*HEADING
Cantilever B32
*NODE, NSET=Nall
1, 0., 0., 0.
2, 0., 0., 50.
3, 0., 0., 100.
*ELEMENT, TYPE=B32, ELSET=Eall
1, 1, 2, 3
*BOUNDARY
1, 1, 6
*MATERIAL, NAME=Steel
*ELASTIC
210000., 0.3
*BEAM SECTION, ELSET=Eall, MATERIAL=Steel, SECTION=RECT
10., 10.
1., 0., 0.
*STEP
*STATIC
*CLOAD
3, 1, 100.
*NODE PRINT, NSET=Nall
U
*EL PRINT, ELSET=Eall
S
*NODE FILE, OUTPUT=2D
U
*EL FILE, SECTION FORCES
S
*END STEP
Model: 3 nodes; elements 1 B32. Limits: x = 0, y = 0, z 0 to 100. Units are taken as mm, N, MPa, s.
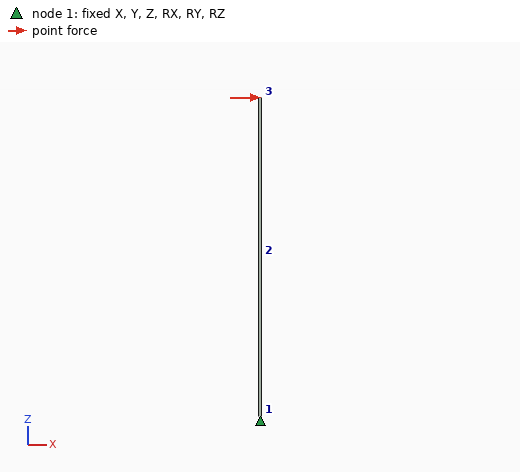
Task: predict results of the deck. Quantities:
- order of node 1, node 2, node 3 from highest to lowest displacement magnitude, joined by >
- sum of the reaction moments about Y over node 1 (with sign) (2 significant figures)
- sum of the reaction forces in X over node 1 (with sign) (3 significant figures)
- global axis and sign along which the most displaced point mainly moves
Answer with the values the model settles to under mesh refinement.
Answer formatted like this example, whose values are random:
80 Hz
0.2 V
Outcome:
node 3 > node 2 > node 1
-10000 N·mm
-100 N
+X
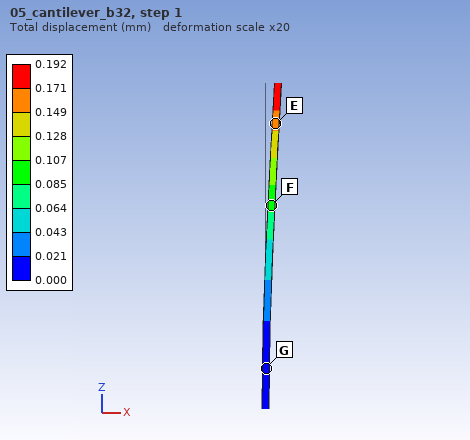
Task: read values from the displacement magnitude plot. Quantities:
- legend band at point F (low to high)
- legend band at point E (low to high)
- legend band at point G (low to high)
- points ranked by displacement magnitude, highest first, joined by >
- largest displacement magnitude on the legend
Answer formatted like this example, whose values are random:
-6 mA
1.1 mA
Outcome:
0.085 to 0.107 mm
0.149 to 0.171 mm
0.000 to 0.021 mm
E > F > G
0.192 mm
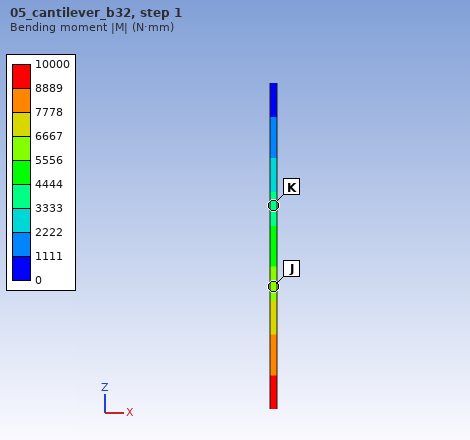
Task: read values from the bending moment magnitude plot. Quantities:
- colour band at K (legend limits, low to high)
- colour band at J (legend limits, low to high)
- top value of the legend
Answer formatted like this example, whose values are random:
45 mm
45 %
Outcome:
3333 to 4444 N·mm
5556 to 6667 N·mm
10000 N·mm
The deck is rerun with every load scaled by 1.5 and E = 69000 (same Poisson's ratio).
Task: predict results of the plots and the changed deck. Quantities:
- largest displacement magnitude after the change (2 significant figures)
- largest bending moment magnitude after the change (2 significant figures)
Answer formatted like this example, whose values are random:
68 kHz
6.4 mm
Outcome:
0.88 mm
15000 N·mm
